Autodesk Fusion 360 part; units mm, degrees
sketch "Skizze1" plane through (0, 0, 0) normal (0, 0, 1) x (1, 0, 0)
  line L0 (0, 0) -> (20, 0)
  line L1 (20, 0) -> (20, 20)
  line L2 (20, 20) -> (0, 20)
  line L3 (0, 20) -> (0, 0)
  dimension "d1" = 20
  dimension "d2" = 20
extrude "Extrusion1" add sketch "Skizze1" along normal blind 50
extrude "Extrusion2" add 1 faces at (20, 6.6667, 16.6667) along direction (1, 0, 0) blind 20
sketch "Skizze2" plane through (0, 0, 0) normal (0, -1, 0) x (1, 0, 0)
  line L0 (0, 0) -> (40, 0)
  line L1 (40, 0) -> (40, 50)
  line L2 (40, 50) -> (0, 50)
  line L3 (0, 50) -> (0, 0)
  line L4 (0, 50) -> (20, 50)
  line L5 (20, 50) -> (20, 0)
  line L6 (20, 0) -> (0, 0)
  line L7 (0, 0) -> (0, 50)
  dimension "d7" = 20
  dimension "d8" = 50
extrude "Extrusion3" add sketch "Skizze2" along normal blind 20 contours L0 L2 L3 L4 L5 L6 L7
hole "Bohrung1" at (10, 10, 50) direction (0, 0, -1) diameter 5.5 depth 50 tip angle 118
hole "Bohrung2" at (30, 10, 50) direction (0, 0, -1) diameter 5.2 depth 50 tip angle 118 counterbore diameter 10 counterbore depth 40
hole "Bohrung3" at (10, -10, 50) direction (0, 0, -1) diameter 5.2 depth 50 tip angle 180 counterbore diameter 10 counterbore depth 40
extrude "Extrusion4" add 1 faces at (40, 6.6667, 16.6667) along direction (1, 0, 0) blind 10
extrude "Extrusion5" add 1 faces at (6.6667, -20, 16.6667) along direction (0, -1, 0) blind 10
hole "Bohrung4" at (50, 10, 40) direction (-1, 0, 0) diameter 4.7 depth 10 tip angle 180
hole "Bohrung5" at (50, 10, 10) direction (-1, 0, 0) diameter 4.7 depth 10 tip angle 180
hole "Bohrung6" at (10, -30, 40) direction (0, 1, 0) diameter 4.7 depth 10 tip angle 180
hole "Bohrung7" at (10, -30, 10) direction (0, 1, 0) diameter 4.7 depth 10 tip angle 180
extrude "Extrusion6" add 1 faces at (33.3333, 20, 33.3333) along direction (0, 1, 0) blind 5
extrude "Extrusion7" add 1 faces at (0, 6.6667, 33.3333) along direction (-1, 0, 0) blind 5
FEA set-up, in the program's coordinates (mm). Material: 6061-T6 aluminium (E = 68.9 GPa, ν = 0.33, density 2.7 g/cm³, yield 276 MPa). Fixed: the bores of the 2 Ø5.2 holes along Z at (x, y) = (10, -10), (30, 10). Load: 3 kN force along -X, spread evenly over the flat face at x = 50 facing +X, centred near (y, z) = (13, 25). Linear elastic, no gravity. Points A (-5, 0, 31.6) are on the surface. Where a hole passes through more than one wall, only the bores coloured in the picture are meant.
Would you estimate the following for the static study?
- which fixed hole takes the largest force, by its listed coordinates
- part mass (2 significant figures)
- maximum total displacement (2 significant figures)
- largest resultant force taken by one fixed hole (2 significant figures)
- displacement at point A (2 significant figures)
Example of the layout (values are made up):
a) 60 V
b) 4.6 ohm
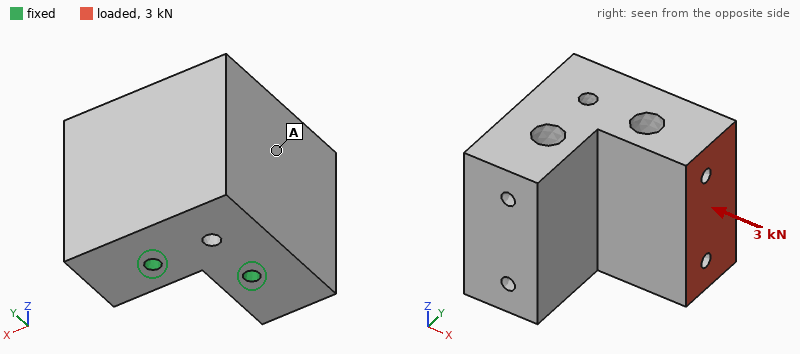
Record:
a) (30, 10)
b) 260 g
c) 42 µm
d) 2.9 kN
e) 23 µm
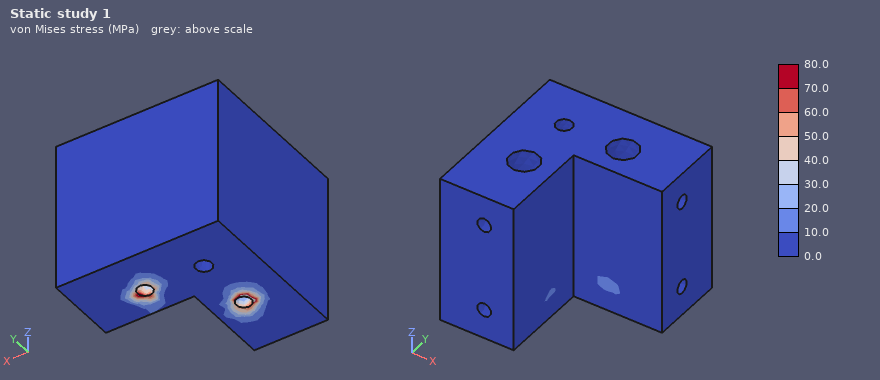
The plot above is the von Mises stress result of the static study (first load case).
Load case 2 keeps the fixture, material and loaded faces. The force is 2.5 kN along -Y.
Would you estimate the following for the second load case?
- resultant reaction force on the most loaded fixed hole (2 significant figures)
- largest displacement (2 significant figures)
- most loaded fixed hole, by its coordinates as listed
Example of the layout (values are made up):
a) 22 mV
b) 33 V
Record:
a) 3.6 kN
b) 51 µm
c) (30, 10)
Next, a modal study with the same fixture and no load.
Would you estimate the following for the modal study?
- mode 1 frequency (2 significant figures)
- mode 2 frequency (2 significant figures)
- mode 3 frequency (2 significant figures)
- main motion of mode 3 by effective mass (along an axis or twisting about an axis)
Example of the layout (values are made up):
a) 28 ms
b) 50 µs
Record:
a) 2800 Hz
b) 5400 Hz
c) 7400 Hz
d) twisting about Z
